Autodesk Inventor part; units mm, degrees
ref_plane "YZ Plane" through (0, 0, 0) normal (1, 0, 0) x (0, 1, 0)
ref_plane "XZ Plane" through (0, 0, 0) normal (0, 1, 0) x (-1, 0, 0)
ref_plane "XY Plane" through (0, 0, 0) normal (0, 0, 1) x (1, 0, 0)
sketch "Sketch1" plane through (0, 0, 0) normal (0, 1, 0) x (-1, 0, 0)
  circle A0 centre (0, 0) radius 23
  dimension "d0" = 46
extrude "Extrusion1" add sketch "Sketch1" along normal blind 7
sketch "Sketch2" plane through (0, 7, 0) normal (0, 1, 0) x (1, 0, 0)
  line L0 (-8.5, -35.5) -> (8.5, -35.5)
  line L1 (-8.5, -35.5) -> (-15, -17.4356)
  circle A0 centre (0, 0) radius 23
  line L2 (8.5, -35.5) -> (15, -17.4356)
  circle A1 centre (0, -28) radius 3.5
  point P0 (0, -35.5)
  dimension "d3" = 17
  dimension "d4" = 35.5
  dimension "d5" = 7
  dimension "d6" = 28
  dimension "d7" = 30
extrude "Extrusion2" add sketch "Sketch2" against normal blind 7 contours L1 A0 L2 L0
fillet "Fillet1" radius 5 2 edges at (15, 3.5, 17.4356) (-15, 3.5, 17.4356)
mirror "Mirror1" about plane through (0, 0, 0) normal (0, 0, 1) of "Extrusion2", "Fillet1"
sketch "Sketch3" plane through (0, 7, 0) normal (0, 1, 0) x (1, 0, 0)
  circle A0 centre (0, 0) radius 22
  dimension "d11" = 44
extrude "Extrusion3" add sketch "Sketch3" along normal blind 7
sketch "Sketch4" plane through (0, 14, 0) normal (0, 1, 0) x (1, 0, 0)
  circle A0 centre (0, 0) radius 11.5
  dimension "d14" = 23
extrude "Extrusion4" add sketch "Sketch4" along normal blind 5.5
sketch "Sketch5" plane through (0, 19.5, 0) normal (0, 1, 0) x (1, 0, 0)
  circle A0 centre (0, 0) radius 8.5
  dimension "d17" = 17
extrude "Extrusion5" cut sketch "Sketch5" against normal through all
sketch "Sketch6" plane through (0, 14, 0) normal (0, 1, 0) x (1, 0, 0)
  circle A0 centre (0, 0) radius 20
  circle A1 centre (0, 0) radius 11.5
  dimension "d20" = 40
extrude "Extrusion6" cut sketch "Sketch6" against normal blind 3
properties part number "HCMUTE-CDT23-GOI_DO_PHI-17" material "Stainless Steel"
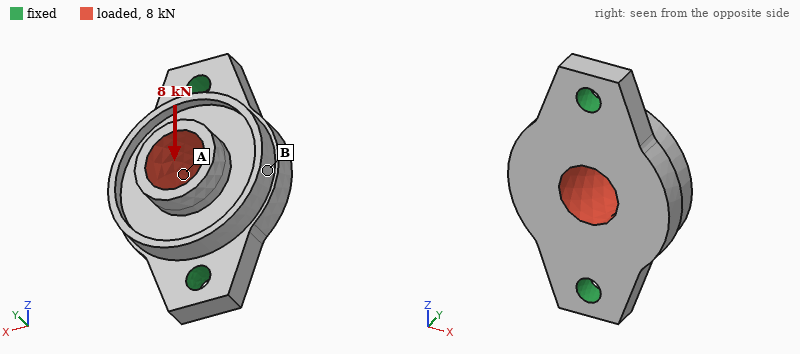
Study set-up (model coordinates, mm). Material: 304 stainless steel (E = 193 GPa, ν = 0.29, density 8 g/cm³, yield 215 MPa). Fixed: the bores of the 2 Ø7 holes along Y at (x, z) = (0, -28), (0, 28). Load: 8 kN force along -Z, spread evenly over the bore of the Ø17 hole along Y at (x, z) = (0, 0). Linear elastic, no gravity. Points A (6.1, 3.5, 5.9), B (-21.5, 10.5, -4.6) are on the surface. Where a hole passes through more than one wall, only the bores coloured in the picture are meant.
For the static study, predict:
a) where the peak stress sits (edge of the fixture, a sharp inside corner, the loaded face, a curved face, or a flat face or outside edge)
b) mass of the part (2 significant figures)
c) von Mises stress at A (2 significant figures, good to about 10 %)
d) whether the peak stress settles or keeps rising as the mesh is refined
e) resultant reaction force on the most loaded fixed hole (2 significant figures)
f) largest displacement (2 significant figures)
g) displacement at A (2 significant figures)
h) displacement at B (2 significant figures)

edge of the fixture
170 g
15 MPa
keeps rising
4.1 kN
7.3 µm
2.3 µm
2.2 µm
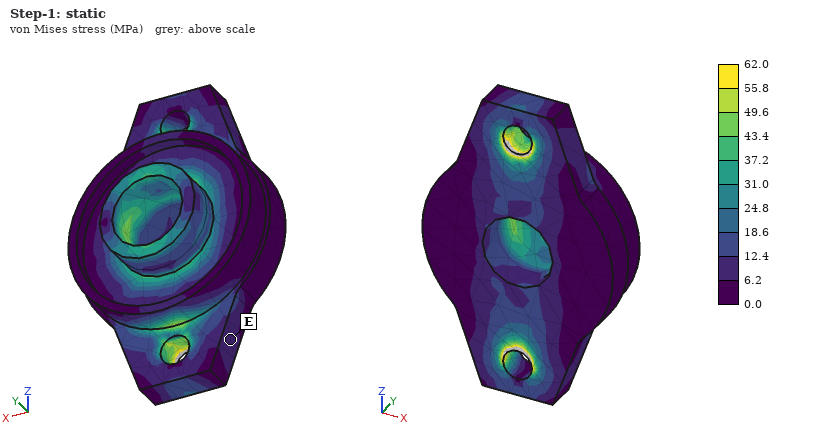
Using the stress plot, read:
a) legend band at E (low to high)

6.2 to 12.4 MPa
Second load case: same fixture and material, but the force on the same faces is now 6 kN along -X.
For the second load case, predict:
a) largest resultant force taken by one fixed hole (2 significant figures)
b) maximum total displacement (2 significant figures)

3.0 kN
23 µm
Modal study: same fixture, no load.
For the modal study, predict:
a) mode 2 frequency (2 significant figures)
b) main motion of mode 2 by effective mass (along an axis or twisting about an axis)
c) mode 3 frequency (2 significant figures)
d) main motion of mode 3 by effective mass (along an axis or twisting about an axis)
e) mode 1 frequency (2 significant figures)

9300 Hz
along Y
18 kHz
along X
6800 Hz
